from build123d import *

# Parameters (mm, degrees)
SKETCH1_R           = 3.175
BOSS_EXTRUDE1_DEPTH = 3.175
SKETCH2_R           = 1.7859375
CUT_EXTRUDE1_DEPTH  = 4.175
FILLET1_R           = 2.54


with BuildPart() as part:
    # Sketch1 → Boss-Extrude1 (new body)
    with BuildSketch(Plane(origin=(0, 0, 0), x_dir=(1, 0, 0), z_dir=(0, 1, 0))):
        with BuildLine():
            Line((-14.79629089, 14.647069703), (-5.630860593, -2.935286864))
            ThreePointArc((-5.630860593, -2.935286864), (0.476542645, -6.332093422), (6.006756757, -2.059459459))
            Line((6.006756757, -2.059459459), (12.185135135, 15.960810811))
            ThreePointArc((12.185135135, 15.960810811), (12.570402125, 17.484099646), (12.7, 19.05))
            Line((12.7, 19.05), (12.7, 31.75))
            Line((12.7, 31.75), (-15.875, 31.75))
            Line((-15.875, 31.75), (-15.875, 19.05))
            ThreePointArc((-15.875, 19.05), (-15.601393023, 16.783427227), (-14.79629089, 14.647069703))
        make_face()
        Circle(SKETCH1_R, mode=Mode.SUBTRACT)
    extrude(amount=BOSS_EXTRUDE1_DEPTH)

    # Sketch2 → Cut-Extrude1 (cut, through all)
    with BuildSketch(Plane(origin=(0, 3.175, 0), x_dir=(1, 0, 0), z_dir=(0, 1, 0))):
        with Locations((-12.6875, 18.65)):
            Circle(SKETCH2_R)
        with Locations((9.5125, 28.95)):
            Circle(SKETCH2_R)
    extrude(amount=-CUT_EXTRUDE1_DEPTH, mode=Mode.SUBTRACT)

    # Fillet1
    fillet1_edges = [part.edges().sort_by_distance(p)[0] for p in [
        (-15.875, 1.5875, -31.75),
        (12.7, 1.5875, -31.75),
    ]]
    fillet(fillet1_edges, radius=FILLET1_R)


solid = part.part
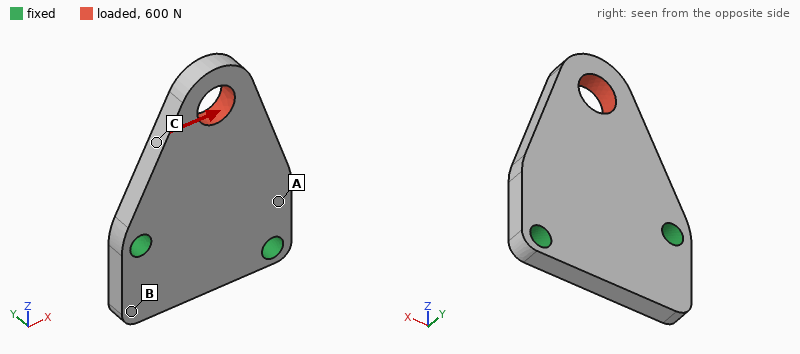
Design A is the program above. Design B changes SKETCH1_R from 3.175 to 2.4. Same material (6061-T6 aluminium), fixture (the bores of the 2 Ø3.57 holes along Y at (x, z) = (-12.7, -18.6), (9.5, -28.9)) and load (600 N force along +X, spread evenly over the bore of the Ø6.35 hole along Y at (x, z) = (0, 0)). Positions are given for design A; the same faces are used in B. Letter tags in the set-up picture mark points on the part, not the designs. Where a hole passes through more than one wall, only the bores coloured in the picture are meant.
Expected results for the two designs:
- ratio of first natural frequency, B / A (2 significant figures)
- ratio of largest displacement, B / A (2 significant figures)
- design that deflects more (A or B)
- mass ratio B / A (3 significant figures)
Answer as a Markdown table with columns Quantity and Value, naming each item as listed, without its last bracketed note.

| Quantity | Value |
|---|---|
| ratio of first natural frequency, B / A | 0.96 |
| ratio of largest displacement, B / A | 0.88 |
| design that deflects more | A |
| mass ratio B / A | 1.02 |
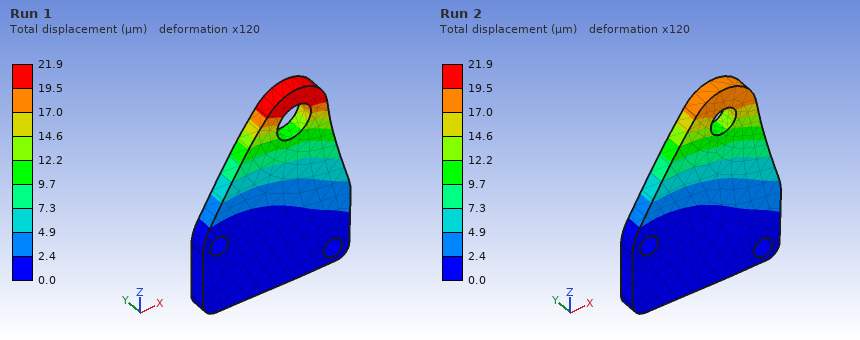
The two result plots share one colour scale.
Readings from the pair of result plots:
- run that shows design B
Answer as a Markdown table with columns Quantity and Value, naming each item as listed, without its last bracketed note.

| Quantity | Value |
|---|---|
| run that shows design B | Run 2 |
